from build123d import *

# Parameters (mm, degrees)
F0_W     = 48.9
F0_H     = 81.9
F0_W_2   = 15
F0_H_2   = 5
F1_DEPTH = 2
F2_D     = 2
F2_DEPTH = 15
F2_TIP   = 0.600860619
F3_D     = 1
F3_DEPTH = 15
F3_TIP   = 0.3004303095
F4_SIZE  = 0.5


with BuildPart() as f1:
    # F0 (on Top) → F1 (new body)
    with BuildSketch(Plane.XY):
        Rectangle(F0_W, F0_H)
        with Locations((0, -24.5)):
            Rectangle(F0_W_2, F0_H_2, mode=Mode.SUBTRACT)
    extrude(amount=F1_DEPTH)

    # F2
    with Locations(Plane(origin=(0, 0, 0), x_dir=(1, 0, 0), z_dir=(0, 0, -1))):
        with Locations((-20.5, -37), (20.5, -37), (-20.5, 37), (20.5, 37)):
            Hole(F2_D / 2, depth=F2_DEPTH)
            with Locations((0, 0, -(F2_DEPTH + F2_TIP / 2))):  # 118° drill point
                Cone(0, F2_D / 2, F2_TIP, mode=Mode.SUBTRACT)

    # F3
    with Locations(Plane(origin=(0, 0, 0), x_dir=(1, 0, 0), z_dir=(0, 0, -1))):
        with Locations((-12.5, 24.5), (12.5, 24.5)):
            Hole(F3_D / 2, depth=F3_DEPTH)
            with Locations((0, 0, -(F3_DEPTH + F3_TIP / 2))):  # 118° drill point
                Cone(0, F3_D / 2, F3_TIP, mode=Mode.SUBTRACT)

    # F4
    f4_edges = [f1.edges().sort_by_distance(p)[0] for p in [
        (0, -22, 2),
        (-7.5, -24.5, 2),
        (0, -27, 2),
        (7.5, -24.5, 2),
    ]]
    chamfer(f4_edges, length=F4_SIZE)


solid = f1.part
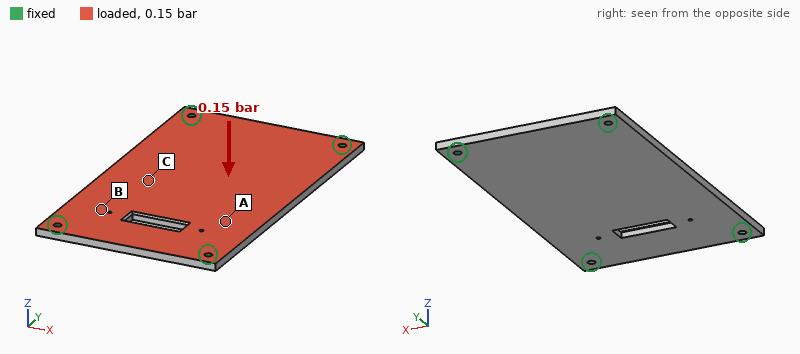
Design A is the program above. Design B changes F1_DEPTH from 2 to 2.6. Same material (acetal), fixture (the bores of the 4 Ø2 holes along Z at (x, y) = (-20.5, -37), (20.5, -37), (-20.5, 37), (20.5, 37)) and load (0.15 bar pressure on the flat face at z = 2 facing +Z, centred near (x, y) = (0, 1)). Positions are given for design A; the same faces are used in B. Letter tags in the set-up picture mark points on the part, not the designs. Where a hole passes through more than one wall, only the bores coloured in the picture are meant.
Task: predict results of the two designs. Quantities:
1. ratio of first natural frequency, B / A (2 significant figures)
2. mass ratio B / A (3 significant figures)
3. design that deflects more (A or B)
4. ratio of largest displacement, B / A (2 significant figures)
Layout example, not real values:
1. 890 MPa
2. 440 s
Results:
1. 1.3
2. 1.30
3. A
4. 0.47
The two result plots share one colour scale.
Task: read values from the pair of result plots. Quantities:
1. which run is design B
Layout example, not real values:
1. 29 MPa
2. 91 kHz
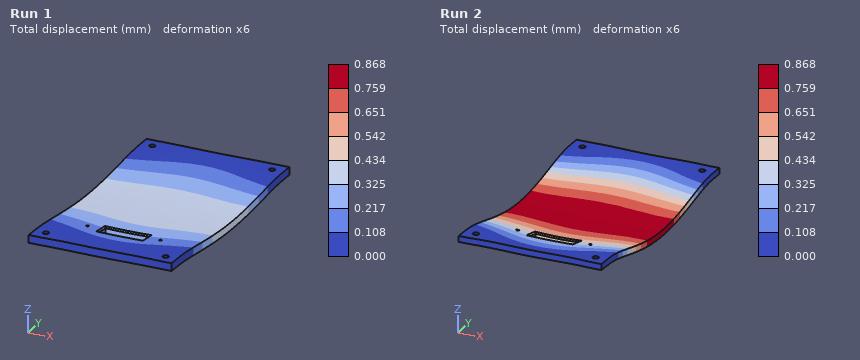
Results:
1. Run 1
